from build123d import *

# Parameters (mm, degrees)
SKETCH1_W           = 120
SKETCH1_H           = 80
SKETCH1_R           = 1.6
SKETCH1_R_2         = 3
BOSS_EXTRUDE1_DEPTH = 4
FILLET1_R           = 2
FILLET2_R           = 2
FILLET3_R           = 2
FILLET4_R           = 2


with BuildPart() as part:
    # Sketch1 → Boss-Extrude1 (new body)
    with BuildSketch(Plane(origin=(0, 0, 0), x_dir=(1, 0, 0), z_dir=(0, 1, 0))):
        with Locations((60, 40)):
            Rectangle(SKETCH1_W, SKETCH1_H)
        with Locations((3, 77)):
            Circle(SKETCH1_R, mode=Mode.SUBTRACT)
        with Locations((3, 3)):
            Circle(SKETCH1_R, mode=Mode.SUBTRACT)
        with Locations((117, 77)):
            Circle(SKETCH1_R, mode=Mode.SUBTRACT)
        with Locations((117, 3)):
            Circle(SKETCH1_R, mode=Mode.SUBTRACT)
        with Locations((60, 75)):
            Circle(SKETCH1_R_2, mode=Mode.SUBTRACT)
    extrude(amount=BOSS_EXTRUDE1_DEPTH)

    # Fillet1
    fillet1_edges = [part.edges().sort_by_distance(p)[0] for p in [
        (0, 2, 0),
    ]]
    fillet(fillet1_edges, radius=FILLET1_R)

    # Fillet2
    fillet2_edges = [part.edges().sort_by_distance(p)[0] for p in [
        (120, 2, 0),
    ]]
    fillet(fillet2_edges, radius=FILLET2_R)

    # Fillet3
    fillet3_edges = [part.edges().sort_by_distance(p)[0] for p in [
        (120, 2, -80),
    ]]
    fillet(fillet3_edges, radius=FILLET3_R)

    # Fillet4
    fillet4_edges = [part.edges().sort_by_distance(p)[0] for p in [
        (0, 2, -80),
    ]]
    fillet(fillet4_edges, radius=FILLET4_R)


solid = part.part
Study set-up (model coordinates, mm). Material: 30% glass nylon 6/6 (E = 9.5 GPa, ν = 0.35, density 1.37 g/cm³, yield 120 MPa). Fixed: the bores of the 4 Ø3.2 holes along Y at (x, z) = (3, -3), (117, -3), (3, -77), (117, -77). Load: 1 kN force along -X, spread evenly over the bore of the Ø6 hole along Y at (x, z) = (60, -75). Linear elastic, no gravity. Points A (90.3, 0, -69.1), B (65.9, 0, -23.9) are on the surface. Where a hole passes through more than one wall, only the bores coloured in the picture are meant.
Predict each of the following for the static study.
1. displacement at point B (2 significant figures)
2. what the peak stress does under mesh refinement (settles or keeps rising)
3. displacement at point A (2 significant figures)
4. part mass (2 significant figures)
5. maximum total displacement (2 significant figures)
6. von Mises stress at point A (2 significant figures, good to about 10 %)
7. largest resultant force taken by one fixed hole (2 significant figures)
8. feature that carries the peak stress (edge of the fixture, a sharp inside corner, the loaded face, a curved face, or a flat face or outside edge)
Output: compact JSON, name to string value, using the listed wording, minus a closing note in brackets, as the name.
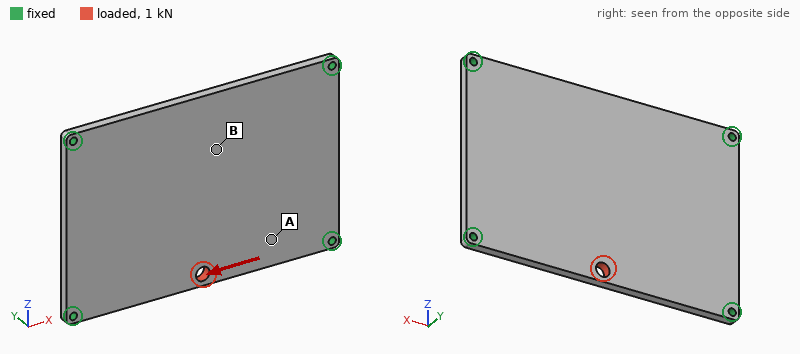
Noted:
{"displacement at point B": "9.6 µm", "what the peak stress does under mesh refinement": "keeps rising", "displacement at point A": "23 µm", "part mass": "52 g", "maximum total displacement": "53 µm", "von Mises stress at point A": "4.3 MPa", "largest resultant force taken by one fixed hole": "340 N", "feature that carries the peak stress": "edge of the fixture"}
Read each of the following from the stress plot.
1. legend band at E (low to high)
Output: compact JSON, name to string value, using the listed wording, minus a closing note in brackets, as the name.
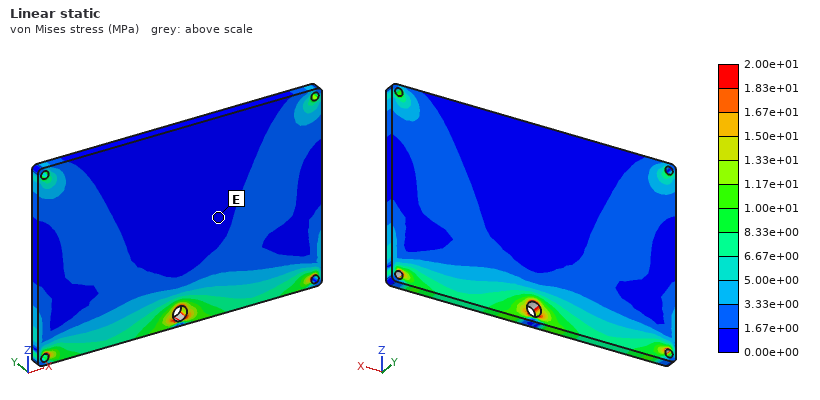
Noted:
{"legend band at E": "0.00e+00 to 1.67e+00 MPa"}
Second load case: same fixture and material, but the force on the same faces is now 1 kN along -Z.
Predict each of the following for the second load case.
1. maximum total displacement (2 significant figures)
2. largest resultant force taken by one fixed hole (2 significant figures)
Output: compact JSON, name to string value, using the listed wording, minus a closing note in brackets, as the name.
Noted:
{"maximum total displacement": "84 µm", "largest resultant force taken by one fixed hole": "330 N"}
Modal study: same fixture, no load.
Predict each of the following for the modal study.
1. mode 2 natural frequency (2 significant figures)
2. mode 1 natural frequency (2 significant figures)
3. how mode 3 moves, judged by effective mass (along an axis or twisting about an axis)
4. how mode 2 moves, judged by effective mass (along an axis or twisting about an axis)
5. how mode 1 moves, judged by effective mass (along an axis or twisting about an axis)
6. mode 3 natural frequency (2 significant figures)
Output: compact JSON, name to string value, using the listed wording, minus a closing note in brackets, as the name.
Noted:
{"mode 2 natural frequency": "1100 Hz", "mode 1 natural frequency": "600 Hz", "how mode 3 moves, judged by effective mass": "twisting about Z", "how mode 2 moves, judged by effective mass": "twisting about X", "how mode 1 moves, judged by effective mass": "along Y", "mode 3 natural frequency": "1500 Hz"}
